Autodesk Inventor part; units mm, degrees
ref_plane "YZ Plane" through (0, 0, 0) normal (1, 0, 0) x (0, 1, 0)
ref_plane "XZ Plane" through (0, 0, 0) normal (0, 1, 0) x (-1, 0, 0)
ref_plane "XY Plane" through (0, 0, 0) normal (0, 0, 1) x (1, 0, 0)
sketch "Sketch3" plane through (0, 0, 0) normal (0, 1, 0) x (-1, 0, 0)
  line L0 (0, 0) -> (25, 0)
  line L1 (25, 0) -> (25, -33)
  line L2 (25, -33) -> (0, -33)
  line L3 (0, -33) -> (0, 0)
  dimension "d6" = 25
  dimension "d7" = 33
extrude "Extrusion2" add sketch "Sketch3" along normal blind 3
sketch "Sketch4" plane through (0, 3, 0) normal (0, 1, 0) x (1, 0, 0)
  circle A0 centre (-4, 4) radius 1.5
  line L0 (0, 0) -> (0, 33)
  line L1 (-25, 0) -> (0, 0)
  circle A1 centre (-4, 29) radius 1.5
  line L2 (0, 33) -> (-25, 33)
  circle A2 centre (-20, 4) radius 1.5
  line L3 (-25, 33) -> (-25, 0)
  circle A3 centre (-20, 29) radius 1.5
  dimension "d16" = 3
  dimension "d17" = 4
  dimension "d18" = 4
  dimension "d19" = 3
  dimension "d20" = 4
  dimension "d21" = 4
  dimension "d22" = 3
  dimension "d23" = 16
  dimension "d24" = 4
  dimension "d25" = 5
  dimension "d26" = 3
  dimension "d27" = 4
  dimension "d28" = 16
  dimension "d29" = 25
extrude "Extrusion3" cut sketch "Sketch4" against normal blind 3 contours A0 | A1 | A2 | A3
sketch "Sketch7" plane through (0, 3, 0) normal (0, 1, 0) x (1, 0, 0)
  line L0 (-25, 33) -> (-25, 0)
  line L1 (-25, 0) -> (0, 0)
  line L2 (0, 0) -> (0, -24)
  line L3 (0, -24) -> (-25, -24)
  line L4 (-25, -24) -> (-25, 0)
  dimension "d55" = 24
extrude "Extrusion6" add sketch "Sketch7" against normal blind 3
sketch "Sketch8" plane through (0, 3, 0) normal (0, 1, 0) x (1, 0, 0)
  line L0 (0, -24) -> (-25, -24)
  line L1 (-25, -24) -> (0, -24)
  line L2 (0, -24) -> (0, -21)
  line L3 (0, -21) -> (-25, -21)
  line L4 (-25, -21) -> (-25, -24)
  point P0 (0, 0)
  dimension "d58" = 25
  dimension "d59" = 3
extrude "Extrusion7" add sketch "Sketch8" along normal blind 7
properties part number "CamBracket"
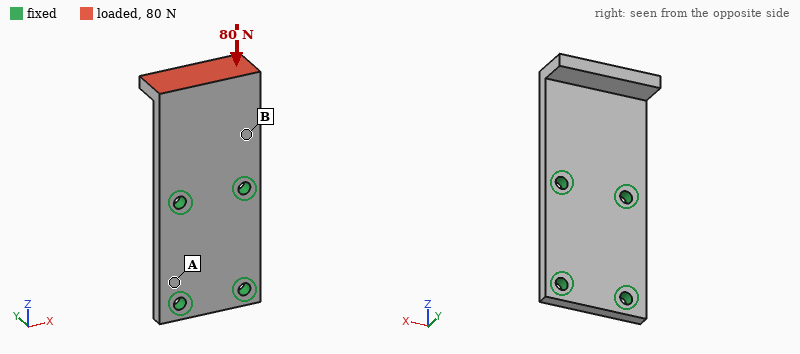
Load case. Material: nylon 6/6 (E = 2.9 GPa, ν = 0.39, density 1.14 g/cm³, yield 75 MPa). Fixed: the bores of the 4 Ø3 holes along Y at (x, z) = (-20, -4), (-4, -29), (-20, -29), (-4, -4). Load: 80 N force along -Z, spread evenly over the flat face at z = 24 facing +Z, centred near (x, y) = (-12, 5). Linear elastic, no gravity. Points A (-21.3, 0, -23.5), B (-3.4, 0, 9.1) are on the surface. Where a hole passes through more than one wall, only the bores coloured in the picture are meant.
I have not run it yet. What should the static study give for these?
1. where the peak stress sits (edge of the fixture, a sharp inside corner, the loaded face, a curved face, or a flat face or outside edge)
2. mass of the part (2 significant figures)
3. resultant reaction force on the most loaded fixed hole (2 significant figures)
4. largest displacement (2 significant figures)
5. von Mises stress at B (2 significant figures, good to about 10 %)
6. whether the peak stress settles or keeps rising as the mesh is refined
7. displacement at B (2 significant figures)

edge of the fixture
5.4 g
39 N
0.74 mm
6.3 MPa
keeps rising
0.13 mm
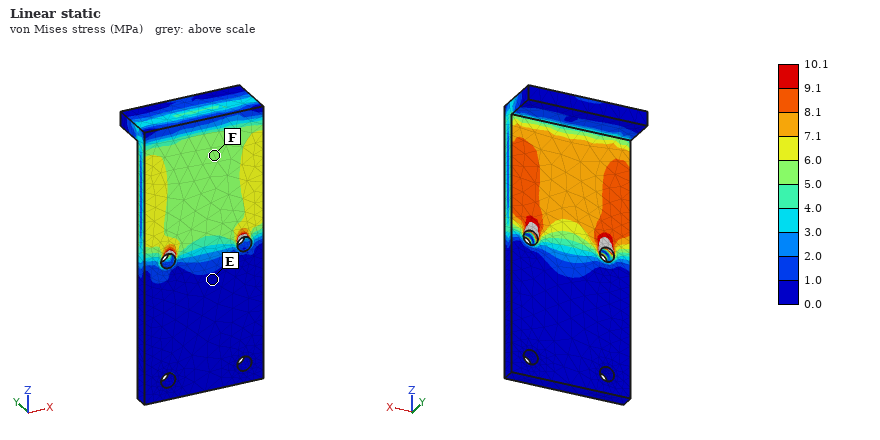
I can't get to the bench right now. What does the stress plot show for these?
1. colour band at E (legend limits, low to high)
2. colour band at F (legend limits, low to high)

0.0 to 1.0 MPa
5.0 to 6.0 MPa
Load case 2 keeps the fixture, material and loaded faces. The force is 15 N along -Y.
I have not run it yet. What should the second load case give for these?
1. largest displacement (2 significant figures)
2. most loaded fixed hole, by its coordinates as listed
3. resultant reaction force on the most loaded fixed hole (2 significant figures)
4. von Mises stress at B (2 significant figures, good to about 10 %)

0.69 mm
(-20, -4)
9.3 N
5.9 MPa
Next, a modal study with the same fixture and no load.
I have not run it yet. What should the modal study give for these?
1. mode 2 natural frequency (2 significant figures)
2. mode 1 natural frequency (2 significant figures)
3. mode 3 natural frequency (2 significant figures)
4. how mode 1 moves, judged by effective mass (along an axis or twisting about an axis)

1800 Hz
730 Hz
4100 Hz
along Y
